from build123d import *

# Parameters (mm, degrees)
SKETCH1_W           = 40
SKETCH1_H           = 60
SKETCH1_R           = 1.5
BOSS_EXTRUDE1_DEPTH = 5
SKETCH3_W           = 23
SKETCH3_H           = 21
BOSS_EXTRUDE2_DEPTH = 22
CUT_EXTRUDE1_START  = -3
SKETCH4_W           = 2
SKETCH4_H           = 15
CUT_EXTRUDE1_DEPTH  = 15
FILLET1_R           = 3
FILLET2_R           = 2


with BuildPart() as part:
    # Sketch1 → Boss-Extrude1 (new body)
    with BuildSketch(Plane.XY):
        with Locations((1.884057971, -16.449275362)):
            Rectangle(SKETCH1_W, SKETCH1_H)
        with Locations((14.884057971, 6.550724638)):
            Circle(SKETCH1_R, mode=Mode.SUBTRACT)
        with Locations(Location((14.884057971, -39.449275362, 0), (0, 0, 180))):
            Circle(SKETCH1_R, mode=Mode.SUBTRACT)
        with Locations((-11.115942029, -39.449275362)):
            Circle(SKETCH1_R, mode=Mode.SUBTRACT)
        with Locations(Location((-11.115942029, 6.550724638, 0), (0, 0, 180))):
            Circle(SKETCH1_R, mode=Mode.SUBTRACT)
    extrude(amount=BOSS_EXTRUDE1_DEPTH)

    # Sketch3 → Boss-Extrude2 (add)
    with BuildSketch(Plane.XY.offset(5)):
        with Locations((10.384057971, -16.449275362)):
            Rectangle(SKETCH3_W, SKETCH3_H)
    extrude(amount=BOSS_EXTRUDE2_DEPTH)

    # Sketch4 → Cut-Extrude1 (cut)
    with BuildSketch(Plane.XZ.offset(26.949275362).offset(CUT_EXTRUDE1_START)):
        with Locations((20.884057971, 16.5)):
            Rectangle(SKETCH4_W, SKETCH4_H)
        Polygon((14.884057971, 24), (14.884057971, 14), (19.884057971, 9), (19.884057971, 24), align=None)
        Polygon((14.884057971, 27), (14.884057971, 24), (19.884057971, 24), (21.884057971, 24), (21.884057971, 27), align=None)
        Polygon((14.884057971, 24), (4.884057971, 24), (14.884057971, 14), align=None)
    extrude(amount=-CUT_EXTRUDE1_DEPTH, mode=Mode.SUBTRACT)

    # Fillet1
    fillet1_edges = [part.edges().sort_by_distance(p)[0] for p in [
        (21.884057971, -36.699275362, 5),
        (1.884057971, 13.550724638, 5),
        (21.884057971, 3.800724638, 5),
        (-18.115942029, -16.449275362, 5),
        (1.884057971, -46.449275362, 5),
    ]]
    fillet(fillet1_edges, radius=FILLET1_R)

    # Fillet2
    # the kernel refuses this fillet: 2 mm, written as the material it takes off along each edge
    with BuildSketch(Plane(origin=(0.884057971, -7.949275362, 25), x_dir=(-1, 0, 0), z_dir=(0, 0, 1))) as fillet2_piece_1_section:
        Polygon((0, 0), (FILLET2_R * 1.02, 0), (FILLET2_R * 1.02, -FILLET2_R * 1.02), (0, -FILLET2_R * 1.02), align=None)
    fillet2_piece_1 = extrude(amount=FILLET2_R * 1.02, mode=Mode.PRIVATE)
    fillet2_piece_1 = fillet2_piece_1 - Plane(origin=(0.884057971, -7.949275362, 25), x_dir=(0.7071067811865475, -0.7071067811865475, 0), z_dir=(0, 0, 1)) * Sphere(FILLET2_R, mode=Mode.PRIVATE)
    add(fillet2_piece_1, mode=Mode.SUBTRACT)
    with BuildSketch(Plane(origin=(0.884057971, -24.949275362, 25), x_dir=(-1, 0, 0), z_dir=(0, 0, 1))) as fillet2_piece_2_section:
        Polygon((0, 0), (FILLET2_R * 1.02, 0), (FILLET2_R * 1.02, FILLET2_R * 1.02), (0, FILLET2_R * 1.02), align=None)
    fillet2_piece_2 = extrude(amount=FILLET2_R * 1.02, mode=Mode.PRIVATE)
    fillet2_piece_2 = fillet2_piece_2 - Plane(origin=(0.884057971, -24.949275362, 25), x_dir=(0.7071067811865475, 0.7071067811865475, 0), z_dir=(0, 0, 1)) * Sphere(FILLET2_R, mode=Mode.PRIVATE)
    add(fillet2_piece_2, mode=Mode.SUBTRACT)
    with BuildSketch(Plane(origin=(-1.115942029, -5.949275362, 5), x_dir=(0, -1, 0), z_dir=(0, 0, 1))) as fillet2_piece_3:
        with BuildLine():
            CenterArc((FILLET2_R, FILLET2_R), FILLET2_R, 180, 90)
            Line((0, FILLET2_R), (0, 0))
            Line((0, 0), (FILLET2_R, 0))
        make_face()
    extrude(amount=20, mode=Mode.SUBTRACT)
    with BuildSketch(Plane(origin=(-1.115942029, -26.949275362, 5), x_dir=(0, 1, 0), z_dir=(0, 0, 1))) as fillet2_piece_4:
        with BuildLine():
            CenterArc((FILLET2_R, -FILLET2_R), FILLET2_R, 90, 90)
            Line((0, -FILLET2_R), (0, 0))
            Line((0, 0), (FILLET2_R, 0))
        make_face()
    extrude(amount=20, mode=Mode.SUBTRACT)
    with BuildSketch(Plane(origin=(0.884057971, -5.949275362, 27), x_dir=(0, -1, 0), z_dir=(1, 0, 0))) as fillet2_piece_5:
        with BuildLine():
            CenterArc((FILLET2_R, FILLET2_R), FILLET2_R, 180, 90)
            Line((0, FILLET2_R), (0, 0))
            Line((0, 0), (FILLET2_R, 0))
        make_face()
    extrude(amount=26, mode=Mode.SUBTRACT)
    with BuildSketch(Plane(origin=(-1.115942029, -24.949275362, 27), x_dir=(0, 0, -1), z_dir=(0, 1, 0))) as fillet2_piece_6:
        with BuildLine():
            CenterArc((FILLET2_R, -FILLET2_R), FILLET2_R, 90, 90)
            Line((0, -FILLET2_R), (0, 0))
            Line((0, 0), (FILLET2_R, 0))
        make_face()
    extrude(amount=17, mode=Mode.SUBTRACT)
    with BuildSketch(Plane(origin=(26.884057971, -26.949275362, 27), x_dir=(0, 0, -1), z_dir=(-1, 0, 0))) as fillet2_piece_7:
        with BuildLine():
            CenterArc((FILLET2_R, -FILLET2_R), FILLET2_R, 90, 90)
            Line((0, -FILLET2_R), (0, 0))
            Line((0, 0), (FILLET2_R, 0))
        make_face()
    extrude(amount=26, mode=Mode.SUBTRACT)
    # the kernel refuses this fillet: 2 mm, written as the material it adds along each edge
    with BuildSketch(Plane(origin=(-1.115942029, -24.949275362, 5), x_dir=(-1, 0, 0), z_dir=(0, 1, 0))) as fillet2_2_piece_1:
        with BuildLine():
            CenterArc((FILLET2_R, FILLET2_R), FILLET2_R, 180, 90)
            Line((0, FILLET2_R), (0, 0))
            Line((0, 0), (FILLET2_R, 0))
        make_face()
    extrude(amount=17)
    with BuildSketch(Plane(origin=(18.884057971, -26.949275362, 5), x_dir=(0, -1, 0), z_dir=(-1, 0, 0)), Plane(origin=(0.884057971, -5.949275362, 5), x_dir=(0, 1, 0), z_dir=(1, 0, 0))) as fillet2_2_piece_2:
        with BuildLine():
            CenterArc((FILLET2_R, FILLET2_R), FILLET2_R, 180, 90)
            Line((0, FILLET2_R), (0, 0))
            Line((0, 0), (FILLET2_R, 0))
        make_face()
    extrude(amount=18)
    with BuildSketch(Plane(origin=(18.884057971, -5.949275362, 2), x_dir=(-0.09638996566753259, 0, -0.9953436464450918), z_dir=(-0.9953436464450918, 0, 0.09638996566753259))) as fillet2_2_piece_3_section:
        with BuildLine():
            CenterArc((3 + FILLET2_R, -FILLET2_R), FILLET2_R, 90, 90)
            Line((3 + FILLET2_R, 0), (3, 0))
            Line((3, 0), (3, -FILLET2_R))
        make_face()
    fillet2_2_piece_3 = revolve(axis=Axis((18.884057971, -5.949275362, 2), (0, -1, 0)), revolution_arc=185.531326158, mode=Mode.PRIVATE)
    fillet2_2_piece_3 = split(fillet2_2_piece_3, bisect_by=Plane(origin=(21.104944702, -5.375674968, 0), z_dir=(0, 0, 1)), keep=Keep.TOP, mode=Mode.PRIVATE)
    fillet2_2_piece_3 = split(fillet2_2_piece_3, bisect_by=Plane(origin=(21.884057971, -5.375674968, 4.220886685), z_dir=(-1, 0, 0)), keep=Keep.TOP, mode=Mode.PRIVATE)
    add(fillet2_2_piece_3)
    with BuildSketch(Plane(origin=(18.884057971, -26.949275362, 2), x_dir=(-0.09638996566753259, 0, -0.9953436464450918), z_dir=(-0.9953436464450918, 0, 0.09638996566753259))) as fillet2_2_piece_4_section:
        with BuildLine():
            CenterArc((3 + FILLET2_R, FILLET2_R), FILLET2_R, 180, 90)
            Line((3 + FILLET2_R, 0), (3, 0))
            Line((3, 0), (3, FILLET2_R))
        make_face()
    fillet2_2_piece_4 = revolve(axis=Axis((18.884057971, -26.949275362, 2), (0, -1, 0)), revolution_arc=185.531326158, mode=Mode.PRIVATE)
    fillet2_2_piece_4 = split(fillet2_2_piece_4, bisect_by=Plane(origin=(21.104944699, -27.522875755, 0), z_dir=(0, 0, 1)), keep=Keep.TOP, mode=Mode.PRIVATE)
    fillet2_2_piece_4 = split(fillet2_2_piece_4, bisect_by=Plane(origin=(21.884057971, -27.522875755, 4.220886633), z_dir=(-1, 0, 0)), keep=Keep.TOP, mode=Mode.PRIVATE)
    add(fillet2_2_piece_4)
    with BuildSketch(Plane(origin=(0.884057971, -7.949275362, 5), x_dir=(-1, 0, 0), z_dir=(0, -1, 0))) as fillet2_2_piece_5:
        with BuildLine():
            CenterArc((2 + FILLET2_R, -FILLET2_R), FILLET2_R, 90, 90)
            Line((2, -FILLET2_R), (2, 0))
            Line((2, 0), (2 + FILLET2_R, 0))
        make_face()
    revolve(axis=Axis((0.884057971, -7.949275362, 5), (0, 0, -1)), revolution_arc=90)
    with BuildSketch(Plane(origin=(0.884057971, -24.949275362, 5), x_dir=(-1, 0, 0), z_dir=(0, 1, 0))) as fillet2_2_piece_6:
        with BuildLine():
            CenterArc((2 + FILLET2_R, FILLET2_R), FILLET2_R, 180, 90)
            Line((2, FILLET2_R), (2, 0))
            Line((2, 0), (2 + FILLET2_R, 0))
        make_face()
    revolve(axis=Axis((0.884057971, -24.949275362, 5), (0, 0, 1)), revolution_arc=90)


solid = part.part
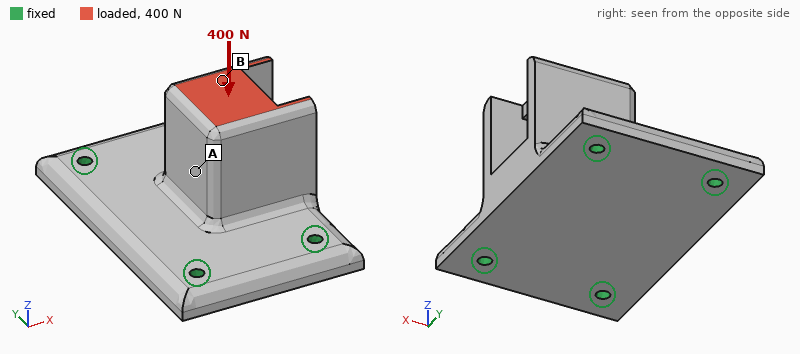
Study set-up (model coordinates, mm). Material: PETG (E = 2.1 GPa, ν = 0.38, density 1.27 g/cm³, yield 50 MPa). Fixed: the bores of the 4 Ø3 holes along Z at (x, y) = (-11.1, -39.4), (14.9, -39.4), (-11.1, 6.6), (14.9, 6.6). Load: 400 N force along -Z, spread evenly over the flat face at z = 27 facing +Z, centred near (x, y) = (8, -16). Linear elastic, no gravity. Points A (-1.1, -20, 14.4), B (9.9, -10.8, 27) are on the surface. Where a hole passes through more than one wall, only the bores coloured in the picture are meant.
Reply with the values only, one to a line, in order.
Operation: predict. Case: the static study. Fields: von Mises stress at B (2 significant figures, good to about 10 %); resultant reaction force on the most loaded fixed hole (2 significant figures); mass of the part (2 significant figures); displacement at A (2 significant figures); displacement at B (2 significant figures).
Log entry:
6.8 MPa
160 N
25 g
0.13 mm
0.19 mm
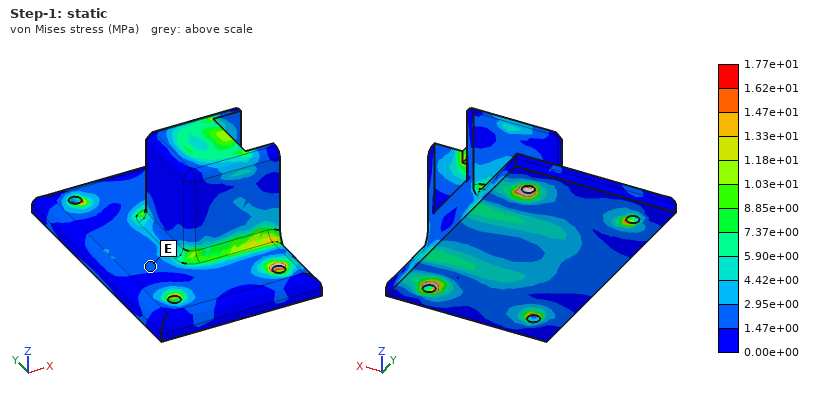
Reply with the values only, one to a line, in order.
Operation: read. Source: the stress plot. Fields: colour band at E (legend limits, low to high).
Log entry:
1.47e+00 to 2.95e+00 MPa
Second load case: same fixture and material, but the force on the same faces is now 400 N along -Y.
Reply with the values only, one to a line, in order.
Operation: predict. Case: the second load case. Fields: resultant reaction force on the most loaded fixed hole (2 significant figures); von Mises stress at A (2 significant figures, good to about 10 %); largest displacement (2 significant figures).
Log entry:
230 N
2.2 MPa
0.50 mm
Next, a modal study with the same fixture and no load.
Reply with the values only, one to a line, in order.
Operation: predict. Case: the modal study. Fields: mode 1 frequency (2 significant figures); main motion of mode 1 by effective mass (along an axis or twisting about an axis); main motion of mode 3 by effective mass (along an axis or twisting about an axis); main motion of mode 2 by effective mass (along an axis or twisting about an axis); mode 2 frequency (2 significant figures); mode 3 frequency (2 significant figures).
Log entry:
1700 Hz
along X
along Y
along Z
2100 Hz
2600 Hz
